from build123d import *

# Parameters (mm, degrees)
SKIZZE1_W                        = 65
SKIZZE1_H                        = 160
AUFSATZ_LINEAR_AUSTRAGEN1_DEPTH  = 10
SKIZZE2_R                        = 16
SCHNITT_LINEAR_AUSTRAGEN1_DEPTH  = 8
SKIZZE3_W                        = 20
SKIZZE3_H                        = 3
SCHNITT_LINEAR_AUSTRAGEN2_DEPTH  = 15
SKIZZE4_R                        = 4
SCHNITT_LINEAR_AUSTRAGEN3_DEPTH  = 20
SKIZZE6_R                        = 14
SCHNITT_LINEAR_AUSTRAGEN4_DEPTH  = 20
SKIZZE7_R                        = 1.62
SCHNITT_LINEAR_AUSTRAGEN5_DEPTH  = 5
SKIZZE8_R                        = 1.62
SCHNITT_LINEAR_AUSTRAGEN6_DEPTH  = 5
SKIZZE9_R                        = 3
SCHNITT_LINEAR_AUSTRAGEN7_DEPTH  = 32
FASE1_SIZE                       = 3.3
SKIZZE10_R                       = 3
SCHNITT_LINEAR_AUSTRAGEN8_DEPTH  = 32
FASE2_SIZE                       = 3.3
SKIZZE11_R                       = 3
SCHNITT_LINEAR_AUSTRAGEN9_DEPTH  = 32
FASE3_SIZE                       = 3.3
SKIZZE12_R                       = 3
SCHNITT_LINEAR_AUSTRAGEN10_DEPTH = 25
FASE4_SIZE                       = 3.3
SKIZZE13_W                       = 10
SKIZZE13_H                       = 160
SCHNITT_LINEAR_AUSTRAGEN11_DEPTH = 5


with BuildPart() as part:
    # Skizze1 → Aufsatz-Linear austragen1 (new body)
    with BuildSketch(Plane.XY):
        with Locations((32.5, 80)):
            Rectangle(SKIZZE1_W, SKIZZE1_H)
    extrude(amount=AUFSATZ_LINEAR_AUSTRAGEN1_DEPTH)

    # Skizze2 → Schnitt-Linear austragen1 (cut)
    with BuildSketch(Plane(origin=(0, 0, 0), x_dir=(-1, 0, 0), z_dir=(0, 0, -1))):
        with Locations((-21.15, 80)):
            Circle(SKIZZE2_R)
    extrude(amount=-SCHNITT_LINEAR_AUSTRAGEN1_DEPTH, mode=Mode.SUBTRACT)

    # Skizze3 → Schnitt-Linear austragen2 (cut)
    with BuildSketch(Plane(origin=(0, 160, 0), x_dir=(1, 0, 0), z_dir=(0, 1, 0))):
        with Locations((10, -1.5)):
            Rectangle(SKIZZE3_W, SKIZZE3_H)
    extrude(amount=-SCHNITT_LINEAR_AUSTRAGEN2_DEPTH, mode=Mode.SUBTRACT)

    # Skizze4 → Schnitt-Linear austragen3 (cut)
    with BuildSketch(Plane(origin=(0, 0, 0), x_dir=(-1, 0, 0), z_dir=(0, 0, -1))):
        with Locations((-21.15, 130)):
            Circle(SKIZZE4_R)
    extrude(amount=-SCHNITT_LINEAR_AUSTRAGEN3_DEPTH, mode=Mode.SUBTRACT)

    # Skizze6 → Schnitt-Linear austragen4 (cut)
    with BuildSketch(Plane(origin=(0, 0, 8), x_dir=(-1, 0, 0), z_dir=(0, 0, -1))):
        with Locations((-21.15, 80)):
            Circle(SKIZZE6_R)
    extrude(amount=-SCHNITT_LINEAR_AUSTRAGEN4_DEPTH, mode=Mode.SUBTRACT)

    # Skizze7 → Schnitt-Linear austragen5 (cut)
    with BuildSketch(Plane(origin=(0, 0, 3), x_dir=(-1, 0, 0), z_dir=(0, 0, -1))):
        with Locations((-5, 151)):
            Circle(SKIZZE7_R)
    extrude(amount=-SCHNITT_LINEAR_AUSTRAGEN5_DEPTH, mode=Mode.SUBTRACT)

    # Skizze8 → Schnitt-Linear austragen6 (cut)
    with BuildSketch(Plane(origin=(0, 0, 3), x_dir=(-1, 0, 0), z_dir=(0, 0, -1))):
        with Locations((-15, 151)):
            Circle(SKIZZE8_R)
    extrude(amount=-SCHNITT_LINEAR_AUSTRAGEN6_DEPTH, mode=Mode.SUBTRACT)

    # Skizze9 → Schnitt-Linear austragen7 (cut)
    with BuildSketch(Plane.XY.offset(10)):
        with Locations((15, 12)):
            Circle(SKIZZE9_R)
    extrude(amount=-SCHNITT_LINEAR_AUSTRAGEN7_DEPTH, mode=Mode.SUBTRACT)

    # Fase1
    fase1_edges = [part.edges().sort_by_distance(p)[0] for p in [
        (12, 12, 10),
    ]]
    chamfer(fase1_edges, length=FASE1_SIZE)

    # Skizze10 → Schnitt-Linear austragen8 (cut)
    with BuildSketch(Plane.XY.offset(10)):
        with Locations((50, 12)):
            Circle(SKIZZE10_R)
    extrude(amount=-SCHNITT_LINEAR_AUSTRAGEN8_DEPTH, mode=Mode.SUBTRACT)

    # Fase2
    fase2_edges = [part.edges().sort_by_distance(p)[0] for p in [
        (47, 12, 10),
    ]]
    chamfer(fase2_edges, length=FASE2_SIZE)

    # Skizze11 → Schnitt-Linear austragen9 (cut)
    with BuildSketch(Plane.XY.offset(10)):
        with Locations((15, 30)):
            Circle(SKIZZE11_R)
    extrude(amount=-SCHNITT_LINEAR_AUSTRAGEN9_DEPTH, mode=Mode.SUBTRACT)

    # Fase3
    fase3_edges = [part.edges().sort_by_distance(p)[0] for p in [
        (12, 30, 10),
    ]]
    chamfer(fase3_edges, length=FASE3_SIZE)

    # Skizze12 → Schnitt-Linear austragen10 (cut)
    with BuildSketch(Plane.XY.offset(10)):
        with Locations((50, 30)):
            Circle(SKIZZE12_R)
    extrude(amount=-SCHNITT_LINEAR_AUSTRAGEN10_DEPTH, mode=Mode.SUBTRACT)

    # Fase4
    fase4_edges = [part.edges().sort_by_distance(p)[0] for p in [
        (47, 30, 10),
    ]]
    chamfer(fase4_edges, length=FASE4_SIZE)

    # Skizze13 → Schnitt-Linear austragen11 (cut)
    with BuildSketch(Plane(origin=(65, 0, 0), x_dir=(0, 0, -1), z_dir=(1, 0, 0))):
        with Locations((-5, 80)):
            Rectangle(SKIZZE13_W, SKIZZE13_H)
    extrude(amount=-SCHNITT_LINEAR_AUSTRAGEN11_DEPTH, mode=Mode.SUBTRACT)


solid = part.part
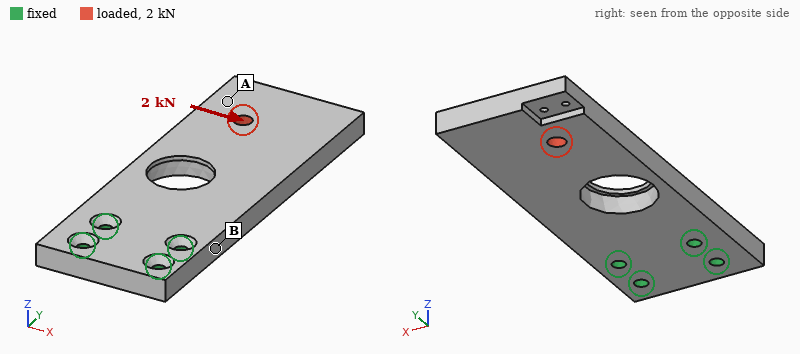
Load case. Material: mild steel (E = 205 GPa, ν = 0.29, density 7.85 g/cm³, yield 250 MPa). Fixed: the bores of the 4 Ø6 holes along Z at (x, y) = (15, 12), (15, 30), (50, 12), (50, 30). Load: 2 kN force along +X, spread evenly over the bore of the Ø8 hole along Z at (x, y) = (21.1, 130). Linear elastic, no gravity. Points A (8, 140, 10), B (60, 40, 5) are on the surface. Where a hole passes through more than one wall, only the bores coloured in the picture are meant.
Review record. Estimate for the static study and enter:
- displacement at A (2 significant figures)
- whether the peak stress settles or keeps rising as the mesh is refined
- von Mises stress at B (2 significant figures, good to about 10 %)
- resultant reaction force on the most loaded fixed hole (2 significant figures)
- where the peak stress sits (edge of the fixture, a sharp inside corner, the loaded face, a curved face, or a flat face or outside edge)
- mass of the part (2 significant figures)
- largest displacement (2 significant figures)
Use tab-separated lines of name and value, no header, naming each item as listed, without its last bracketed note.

displacement at A	41 µm
whether the peak stress settles or keeps rising as the mesh is refined	keeps rising
von Mises stress at B	31 MPa
resultant reaction force on the most loaded fixed hole	4.2 kN
where the peak stress sits	edge of the fixture
mass of the part	670 g
largest displacement	50 µm
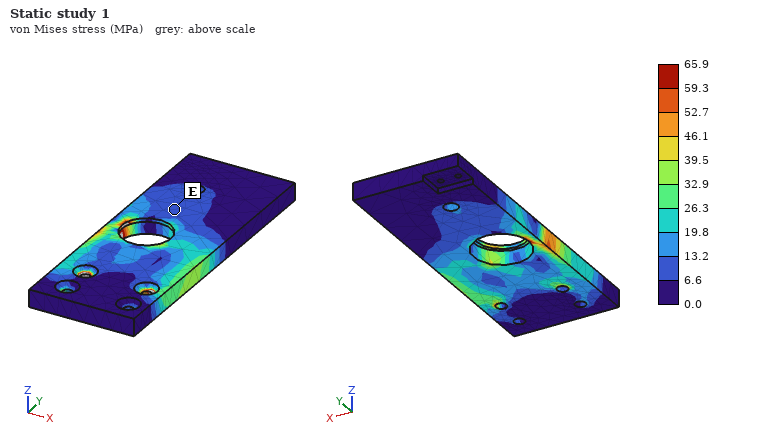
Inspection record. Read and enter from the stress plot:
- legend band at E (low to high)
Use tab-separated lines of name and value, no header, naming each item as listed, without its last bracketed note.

legend band at E	6.6 to 13.2 MPa
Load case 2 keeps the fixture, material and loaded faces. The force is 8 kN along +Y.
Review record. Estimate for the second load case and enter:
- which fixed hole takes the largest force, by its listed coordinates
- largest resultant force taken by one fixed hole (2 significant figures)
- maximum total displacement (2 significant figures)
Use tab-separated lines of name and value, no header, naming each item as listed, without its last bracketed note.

which fixed hole takes the largest force, by its listed coordinates	(15, 30)
largest resultant force taken by one fixed hole	4.6 kN
maximum total displacement	41 µm
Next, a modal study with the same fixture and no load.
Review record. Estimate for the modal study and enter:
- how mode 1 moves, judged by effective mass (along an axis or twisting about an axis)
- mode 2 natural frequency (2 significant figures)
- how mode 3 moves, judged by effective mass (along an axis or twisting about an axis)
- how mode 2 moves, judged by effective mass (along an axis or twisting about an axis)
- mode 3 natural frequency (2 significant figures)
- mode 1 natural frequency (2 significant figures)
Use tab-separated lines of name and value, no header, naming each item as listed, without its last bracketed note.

how mode 1 moves, judged by effective mass	along Z
mode 2 natural frequency	1900 Hz
how mode 3 moves, judged by effective mass	along X
how mode 2 moves, judged by effective mass	twisting about Y
mode 3 natural frequency	2100 Hz
mode 1 natural frequency	430 Hz
